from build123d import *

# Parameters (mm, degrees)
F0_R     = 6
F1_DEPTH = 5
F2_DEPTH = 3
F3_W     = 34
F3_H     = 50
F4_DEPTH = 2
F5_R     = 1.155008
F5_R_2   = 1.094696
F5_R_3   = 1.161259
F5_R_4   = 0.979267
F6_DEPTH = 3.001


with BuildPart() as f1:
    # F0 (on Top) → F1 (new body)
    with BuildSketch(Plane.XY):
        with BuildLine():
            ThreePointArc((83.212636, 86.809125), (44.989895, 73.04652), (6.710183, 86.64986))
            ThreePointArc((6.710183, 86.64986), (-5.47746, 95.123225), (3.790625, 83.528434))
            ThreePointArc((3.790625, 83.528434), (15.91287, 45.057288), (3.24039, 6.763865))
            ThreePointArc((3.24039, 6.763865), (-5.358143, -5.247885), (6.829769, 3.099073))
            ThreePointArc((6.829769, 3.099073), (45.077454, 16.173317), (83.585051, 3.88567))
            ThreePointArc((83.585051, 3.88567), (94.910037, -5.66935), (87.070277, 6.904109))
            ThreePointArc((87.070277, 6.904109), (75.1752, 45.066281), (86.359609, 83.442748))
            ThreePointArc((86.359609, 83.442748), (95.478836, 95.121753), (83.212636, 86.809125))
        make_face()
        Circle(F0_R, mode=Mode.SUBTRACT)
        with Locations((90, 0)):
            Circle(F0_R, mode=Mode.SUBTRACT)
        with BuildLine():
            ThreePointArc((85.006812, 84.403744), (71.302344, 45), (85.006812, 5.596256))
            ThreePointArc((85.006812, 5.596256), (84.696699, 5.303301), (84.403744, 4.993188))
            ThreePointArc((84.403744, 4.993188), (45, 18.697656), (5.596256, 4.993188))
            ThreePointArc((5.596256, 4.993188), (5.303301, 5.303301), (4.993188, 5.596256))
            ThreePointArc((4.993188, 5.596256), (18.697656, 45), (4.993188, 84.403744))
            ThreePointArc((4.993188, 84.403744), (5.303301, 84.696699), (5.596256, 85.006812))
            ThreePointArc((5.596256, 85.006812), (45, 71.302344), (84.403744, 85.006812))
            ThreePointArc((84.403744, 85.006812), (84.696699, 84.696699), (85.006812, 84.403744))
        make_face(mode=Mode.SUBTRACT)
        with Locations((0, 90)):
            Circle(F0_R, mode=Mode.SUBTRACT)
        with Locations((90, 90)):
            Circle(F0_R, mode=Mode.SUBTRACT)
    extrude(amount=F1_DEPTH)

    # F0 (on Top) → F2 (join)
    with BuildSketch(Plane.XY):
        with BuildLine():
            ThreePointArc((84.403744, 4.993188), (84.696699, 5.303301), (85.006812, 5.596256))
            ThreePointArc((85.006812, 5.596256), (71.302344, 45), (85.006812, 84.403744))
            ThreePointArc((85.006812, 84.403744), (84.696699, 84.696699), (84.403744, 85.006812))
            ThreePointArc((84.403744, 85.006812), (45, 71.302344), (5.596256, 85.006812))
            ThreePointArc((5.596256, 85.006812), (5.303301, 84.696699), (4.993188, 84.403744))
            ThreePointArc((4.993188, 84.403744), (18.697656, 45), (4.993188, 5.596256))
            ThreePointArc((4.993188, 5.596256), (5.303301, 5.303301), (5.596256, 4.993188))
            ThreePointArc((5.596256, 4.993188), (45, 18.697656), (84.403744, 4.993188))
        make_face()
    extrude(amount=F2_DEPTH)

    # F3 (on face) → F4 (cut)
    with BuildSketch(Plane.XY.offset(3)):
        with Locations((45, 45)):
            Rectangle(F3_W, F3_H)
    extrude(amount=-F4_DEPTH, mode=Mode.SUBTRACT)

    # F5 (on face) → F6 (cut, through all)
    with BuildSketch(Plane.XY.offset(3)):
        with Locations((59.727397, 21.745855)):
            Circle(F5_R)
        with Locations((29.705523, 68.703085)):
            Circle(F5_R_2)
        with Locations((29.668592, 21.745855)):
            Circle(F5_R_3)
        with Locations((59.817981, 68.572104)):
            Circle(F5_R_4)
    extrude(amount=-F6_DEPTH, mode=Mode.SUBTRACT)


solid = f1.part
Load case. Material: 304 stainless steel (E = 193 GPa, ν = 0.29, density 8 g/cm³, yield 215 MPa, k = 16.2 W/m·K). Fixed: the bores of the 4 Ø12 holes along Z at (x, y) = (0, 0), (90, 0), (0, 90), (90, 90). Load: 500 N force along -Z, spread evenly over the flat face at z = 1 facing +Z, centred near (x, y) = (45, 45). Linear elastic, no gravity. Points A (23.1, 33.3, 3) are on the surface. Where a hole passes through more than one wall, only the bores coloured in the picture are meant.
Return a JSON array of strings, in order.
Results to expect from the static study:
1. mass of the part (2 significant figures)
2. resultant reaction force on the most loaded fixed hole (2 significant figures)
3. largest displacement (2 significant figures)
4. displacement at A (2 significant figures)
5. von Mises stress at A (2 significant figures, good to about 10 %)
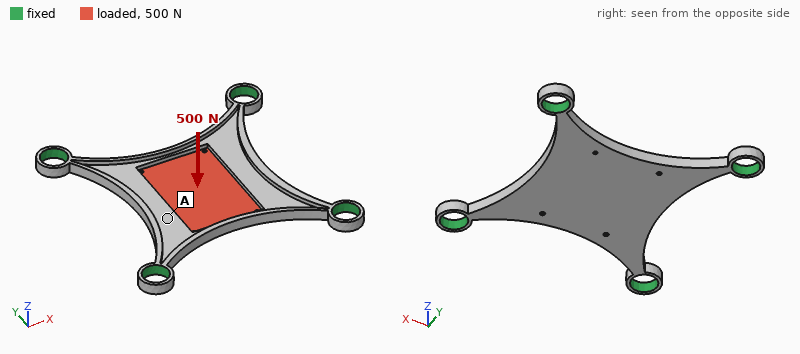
["99 g", "590 N", "0.18 mm", "0.074 mm", "40 MPa"]
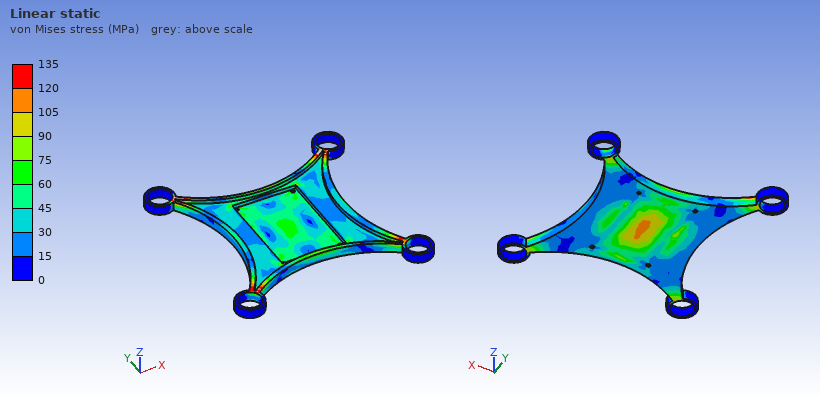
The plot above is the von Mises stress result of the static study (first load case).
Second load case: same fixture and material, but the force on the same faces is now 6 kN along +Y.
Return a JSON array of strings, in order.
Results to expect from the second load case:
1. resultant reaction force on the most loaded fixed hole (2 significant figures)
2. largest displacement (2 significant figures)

["2.0 kN", "28 µm"]
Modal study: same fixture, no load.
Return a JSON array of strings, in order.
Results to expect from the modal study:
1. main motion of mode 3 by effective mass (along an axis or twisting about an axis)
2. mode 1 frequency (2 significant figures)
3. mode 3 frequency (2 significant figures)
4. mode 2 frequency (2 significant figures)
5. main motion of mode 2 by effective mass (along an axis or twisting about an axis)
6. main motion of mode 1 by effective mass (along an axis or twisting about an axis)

["twisting about X", "1800 Hz", "3400 Hz", "2700 Hz", "twisting about Y", "along Z"]
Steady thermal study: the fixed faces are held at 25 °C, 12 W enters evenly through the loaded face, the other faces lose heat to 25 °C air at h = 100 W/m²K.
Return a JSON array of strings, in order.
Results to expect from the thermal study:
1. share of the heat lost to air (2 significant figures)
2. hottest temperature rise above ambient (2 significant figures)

["96 %", "42 K"]
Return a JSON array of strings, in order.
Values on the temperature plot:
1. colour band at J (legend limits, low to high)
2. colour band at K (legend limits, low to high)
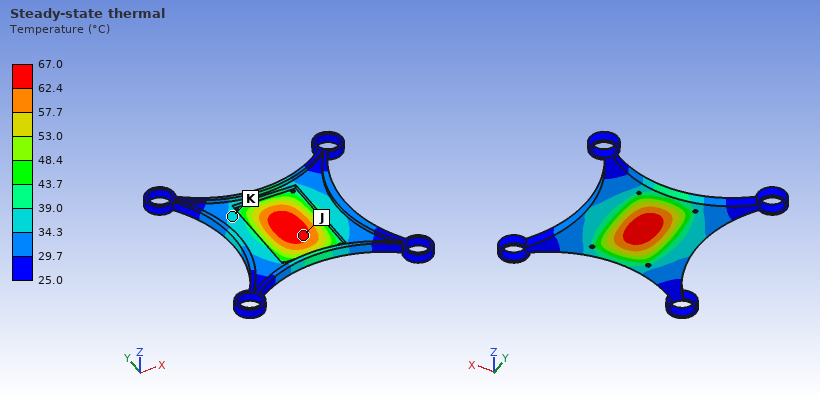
["62.4 to 67.0 °C", "34.3 to 39.0 °C"]
